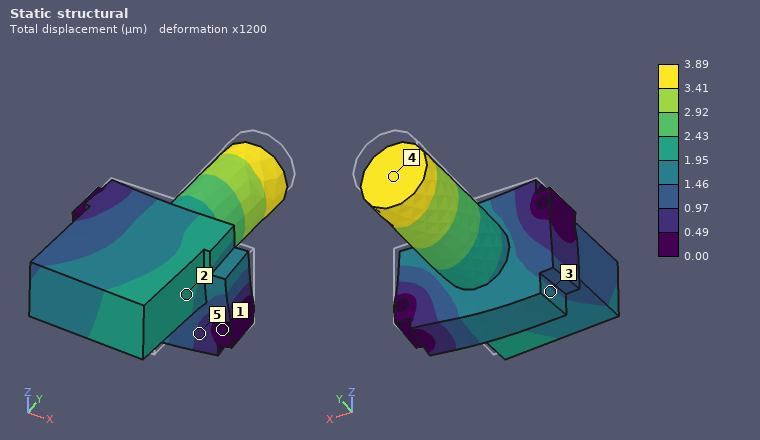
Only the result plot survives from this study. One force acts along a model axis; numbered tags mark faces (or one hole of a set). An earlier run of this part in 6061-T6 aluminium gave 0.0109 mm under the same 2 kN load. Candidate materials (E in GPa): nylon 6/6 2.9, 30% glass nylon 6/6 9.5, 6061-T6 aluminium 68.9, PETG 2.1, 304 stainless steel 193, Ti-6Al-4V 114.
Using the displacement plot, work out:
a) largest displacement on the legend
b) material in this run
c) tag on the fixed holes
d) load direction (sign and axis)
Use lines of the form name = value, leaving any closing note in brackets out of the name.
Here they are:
largest displacement on the legend = 3.89 µm
material in this run = 304 stainless steel
tag on the fixed holes = 1
load direction = -Y
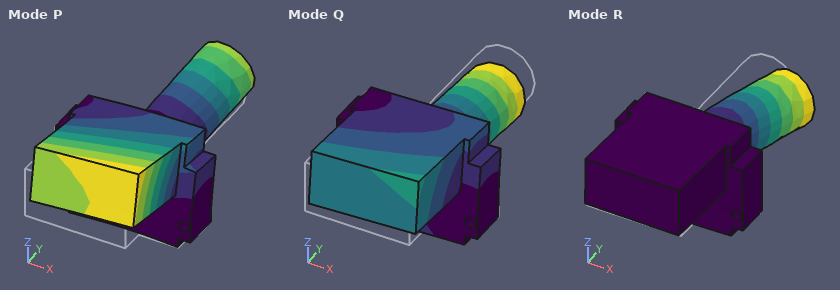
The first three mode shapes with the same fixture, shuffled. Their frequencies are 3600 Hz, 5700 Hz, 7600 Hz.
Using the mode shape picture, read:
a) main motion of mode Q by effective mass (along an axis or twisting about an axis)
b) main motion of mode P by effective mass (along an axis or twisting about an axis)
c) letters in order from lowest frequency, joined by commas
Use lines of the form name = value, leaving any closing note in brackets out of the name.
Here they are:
main motion of mode Q by effective mass = twisting about X
main motion of mode P by effective mass = along Z
letters in order from lowest frequency, joined by commas = Q, R, P
